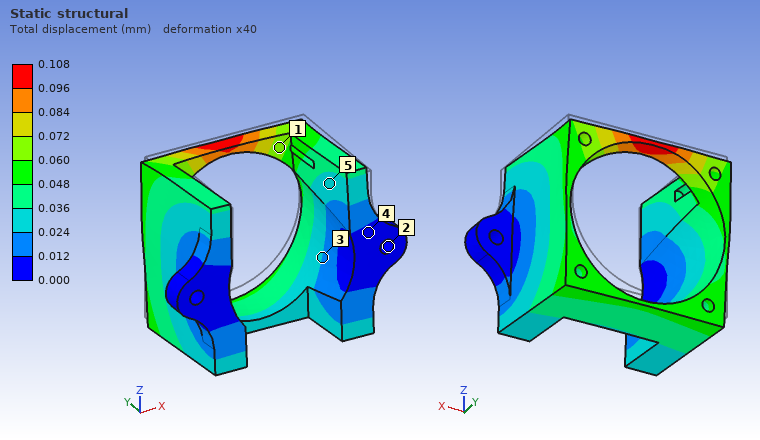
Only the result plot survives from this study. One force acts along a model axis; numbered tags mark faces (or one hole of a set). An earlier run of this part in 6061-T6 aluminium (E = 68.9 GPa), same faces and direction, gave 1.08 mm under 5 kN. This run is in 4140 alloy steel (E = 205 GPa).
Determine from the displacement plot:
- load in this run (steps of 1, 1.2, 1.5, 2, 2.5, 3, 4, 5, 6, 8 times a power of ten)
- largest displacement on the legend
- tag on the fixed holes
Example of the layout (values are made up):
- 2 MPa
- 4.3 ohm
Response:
- 1.5 kN
- 0.108 mm
- 2
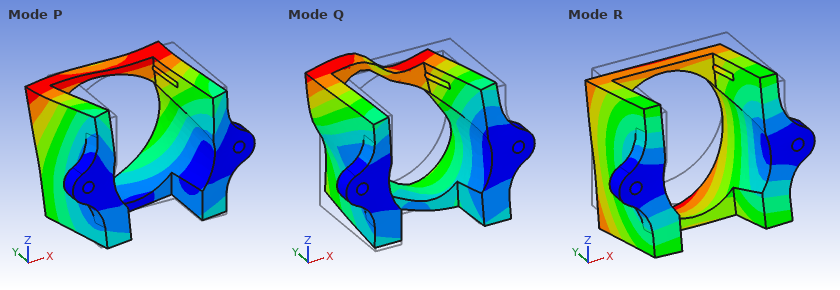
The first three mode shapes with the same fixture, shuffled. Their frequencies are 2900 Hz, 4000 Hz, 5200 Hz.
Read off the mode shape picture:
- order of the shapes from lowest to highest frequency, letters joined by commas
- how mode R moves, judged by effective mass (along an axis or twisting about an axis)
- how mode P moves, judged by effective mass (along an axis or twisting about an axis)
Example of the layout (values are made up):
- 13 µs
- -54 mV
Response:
- R, P, Q
- along Z
- along X
